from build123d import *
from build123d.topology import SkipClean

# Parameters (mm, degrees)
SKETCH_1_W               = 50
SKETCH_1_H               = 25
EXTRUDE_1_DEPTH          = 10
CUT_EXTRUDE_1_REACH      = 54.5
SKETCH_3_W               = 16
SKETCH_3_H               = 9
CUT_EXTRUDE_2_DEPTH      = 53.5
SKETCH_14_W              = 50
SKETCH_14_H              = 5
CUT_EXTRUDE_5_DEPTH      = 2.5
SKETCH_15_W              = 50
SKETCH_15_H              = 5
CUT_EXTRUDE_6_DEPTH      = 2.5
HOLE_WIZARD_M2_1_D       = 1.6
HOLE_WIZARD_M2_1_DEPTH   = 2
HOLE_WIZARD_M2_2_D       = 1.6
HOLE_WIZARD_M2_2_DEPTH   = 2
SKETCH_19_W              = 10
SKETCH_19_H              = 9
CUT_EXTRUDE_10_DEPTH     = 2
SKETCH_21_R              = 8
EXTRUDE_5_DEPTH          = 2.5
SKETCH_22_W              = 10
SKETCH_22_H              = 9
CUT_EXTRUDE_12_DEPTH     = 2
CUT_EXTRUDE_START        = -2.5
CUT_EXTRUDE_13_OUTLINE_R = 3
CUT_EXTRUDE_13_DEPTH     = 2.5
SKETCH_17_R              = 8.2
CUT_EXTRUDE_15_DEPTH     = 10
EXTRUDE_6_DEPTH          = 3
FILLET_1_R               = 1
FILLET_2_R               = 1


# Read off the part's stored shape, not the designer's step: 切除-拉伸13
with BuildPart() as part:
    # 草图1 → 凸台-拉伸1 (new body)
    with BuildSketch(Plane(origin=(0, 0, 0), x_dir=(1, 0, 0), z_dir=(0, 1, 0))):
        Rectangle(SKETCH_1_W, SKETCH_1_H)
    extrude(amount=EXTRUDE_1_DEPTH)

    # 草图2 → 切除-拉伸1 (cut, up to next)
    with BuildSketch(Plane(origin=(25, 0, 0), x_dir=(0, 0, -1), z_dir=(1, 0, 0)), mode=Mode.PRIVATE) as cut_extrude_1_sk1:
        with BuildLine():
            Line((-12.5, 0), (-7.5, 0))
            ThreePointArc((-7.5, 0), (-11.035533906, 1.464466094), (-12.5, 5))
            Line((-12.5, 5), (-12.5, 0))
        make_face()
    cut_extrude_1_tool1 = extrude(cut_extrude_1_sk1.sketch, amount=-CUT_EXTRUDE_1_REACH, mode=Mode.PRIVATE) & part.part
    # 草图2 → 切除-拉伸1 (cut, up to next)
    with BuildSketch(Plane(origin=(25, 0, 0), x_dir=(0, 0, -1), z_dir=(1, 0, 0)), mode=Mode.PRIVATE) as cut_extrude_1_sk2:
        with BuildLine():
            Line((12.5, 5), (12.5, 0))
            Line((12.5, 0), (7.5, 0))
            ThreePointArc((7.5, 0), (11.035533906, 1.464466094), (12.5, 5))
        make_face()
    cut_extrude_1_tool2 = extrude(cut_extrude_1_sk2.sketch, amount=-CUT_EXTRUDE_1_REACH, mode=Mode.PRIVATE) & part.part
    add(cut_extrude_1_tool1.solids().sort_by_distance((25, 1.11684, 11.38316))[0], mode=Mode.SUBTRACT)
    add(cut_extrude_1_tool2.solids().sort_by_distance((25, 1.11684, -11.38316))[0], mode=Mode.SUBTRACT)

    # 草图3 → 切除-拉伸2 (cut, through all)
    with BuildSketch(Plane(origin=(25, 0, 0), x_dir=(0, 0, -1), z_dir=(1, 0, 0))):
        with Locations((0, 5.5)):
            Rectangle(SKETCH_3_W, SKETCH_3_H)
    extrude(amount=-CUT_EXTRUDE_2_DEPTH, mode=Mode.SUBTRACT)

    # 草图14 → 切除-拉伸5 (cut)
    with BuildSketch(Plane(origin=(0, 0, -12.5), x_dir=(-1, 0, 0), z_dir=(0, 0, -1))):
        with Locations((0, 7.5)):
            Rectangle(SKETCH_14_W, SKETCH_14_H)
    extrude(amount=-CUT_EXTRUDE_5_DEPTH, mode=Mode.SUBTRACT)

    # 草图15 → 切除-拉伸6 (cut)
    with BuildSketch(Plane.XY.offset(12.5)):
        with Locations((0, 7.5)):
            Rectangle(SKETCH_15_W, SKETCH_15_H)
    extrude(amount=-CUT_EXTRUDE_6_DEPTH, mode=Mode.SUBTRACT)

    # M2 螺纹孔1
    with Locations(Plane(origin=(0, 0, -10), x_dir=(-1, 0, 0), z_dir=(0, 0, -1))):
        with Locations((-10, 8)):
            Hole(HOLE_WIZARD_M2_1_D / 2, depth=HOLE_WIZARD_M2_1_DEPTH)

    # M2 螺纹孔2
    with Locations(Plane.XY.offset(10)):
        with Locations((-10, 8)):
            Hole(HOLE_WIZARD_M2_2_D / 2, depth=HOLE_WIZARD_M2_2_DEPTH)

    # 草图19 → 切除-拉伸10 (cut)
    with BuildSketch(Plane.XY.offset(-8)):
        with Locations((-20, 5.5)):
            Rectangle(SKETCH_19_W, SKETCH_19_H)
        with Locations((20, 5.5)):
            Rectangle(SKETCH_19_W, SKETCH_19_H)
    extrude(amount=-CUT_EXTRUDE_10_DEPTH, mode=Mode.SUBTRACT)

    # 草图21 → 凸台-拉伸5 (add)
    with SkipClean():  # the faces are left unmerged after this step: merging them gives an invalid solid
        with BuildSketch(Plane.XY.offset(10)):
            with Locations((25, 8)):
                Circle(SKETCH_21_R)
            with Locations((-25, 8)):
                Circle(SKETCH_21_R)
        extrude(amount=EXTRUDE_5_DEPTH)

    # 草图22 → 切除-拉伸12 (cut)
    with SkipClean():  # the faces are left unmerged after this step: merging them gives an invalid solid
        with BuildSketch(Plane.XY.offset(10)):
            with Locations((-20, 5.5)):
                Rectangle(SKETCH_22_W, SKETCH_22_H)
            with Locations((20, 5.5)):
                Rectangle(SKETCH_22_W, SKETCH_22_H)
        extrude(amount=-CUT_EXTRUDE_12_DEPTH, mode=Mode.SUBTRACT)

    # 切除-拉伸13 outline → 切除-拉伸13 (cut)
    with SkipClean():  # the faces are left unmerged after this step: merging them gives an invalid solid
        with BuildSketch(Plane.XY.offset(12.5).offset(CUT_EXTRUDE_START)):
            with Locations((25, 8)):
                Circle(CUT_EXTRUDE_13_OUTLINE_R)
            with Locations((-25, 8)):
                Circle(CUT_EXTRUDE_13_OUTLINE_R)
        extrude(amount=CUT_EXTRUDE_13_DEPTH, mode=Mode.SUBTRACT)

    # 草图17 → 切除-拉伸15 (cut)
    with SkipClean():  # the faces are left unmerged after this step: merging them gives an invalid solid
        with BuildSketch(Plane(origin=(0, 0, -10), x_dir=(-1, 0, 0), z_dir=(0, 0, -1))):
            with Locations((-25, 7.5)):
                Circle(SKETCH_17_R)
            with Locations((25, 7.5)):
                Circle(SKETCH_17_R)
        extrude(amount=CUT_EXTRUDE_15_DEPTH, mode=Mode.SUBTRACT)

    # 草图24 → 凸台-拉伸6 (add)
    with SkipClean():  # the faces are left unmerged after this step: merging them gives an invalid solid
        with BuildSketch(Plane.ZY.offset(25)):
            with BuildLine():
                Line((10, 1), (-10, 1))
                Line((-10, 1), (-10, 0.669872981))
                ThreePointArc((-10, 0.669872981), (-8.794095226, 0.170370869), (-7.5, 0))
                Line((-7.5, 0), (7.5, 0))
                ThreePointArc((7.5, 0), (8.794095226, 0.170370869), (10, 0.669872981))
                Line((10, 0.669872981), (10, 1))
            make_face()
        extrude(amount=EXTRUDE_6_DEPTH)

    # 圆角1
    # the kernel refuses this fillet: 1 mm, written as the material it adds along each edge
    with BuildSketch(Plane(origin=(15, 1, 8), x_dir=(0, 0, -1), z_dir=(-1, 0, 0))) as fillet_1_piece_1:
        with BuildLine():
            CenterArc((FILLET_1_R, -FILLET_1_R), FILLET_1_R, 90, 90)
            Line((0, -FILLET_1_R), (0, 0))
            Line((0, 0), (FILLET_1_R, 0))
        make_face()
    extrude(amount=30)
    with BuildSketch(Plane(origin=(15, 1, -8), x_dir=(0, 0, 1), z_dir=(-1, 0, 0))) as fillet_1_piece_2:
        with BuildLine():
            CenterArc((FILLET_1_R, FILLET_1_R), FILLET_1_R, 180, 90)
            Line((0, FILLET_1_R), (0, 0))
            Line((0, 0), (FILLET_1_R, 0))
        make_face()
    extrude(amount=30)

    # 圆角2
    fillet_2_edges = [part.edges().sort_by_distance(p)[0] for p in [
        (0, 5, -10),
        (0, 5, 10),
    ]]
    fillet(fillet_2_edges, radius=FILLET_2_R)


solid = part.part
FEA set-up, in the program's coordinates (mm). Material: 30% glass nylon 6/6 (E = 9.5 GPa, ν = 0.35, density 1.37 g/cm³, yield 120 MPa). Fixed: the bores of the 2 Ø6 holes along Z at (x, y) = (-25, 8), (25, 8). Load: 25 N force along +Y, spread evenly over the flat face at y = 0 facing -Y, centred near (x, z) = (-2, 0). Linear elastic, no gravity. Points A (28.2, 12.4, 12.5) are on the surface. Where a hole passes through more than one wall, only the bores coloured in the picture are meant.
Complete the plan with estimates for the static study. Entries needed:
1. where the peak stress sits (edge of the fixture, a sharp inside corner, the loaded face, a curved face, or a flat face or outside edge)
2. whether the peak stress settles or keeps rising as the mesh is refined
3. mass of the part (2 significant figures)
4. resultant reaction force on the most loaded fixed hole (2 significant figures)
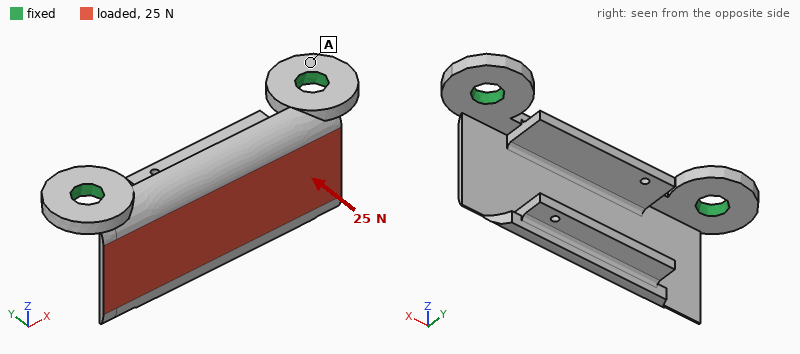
a sharp inside corner
keeps rising
4.8 g
15 N
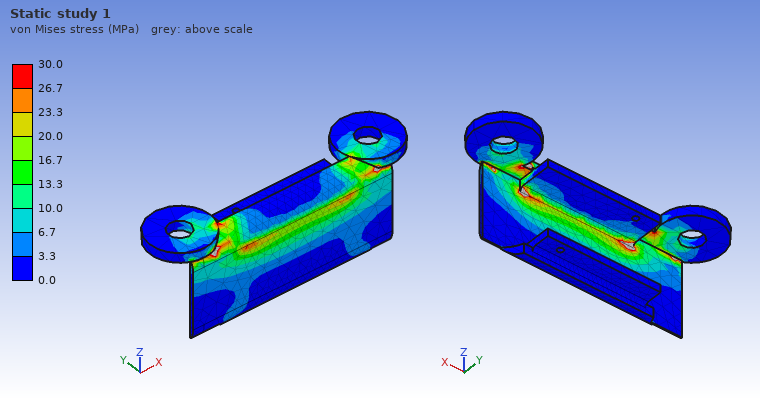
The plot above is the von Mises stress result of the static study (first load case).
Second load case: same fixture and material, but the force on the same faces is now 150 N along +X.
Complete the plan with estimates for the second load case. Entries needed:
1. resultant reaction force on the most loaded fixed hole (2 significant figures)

85 N
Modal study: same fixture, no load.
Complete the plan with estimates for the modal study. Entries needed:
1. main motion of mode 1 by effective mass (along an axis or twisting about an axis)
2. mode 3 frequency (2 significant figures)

along Y
2200 Hz
